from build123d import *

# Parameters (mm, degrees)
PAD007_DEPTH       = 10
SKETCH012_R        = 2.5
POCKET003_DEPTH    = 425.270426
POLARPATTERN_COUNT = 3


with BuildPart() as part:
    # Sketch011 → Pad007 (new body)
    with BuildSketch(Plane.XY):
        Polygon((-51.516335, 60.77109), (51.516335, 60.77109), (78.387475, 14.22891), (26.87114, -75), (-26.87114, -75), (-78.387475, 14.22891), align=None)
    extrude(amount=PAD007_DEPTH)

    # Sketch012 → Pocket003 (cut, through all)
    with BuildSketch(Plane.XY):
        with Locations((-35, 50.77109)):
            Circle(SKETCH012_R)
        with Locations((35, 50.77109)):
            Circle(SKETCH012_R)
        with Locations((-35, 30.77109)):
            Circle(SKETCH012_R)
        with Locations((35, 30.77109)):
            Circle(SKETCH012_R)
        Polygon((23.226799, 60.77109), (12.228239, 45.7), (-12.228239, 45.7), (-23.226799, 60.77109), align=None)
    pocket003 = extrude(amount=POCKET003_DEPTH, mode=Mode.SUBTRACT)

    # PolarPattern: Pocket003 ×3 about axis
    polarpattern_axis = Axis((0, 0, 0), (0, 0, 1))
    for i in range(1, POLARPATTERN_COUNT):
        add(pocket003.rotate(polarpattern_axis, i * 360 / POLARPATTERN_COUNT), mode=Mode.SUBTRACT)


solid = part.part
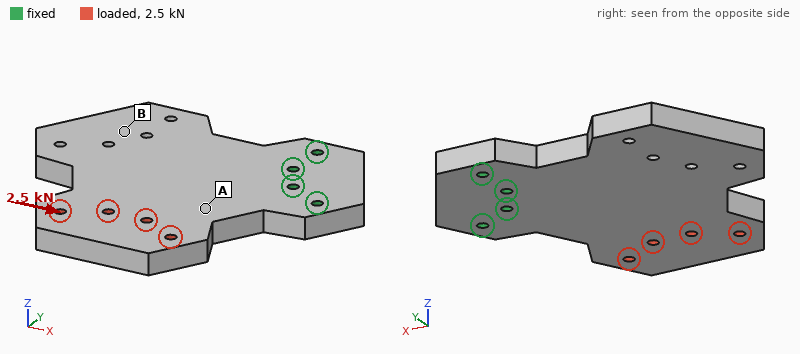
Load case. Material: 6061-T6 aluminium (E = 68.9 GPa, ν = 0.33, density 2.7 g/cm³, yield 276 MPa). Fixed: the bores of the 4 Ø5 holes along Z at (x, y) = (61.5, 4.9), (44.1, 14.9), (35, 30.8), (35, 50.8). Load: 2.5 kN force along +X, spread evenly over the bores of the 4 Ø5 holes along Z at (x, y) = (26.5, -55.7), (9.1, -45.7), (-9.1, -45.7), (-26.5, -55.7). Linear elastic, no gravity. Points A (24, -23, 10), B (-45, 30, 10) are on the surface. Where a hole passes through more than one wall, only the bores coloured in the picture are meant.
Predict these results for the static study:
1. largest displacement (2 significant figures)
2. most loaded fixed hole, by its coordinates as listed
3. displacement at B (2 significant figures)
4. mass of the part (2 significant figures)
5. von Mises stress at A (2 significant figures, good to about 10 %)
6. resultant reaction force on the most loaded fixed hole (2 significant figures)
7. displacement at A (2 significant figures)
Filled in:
57 µm
(61.5, 4.9)
34 µm
370 g
10 MPa
3.3 kN
19 µm
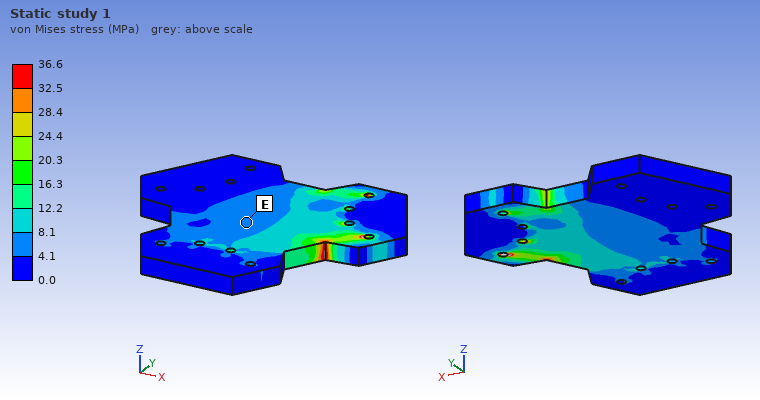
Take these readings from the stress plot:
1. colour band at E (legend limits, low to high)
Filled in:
4.1 to 8.1 MPa
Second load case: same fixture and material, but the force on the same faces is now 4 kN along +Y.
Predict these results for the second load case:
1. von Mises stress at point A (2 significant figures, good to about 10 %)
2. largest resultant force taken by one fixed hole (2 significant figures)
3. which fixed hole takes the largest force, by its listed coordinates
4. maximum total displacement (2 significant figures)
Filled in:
7.1 MPa
2.9 kN
(35, 50.8)
46 µm
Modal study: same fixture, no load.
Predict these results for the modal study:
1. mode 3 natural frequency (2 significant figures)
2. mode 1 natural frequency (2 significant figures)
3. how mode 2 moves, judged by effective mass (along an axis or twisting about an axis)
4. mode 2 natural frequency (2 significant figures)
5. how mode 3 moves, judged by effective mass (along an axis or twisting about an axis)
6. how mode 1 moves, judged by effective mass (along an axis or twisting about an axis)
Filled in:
2600 Hz
600 Hz
twisting about X
950 Hz
along Y
along Z
